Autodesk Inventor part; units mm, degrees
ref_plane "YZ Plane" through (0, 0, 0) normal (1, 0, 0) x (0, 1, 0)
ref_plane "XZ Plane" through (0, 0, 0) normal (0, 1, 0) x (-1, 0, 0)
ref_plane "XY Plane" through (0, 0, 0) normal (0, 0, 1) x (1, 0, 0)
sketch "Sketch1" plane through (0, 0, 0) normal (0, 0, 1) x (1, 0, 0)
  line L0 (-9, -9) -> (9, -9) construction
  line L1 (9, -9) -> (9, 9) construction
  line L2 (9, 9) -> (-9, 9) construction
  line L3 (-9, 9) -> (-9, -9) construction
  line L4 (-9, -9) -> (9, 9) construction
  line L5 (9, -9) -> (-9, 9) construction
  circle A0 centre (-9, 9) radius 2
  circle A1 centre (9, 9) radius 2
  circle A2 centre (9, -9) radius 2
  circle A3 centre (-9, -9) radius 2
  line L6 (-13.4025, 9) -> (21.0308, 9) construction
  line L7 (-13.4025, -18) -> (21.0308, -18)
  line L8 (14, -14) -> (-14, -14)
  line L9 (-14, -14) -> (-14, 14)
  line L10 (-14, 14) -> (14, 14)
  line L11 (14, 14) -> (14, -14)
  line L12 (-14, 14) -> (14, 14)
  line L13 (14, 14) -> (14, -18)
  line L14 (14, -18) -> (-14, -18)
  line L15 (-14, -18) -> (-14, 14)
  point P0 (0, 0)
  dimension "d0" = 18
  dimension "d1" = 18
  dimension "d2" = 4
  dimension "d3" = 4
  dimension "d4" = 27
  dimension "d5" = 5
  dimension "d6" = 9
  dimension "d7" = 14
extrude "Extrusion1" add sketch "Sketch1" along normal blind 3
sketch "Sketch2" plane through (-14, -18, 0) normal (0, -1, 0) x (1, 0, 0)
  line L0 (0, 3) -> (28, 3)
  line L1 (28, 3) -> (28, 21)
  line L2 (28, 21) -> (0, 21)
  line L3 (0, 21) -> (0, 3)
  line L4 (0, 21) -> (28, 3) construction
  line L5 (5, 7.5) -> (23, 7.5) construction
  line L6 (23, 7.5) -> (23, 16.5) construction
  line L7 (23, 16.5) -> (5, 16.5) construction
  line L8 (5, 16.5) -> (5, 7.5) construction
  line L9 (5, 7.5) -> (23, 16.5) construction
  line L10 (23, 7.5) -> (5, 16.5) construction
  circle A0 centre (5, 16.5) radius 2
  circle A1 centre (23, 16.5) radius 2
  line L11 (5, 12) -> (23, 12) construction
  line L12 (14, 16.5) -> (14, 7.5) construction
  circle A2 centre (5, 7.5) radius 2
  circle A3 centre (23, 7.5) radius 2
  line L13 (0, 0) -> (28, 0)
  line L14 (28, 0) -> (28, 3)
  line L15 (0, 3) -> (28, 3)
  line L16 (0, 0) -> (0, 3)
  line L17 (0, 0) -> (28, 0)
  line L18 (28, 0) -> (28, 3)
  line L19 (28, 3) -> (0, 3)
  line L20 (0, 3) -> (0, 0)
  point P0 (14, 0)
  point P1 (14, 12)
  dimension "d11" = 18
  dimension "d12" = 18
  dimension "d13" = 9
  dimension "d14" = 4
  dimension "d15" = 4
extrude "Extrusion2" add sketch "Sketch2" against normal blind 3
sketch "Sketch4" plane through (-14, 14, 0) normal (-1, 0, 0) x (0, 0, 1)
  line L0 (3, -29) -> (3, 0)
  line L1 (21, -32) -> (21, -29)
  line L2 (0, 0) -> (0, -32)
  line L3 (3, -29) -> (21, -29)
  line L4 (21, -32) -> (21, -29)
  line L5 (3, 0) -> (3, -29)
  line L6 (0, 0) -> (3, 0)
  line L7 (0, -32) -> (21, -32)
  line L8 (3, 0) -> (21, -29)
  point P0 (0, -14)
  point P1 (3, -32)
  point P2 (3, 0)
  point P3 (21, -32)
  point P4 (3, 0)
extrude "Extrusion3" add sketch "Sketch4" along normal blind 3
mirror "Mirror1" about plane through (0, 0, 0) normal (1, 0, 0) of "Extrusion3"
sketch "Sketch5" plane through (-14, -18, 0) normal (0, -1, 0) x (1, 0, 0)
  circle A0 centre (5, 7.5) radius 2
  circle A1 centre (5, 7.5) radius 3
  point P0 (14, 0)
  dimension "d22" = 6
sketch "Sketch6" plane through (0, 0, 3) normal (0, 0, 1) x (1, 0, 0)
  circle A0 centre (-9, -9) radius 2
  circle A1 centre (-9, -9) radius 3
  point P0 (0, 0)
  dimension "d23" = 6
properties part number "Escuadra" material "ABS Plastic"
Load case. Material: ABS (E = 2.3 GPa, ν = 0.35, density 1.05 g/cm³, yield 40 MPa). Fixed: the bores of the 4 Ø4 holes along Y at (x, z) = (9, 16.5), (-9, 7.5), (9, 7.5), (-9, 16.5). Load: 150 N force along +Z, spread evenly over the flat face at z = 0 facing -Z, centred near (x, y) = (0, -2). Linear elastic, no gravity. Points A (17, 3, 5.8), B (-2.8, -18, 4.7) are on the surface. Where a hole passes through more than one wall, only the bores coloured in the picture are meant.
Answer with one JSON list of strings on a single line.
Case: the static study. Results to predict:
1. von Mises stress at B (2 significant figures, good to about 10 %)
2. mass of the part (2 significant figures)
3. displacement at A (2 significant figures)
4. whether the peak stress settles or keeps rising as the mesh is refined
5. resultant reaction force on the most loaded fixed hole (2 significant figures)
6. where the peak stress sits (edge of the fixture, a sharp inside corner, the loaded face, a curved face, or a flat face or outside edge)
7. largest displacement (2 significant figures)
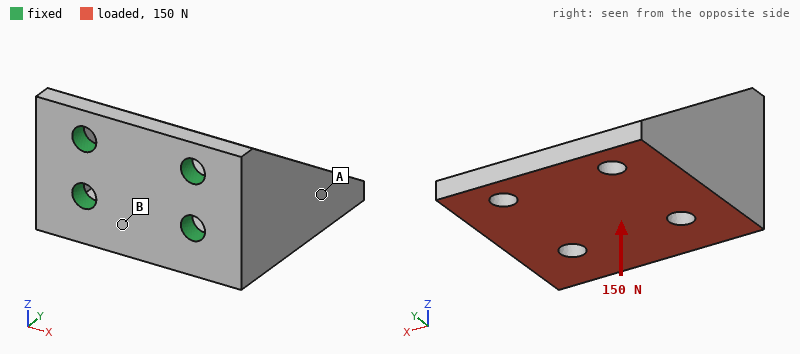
["5.8 MPa", "6.7 g", "0.19 mm", "keeps rising", "91 N", "edge of the fixture", "0.57 mm"]
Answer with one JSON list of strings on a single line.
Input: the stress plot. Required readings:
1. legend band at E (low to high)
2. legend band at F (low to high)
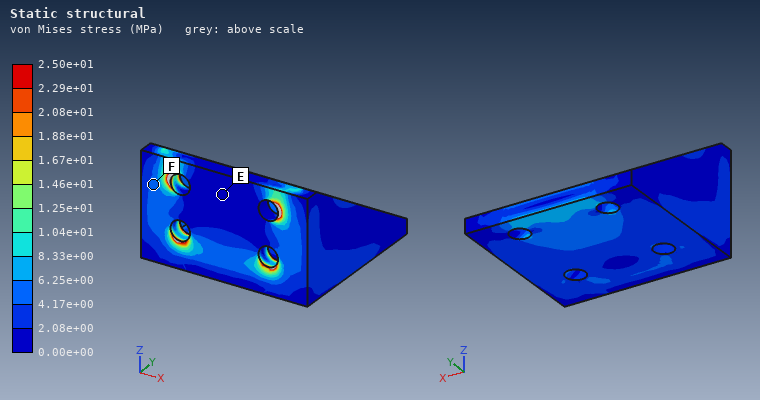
["0.00e+00 to 2.08e+00 MPa", "4.17e+00 to 6.25e+00 MPa"]
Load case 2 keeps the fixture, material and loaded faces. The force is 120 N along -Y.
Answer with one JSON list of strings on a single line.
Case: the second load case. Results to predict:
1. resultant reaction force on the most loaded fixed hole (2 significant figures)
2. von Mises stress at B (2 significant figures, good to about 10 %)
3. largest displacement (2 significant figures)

["80 N", "2.3 MPa", "0.17 mm"]
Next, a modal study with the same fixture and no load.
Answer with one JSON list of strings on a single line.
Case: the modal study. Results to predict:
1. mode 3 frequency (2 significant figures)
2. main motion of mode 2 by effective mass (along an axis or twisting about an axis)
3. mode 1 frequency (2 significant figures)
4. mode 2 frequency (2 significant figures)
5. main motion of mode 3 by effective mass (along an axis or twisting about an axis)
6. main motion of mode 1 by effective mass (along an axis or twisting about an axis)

["3800 Hz", "along X", "1700 Hz", "2000 Hz", "along X", "along Z"]
